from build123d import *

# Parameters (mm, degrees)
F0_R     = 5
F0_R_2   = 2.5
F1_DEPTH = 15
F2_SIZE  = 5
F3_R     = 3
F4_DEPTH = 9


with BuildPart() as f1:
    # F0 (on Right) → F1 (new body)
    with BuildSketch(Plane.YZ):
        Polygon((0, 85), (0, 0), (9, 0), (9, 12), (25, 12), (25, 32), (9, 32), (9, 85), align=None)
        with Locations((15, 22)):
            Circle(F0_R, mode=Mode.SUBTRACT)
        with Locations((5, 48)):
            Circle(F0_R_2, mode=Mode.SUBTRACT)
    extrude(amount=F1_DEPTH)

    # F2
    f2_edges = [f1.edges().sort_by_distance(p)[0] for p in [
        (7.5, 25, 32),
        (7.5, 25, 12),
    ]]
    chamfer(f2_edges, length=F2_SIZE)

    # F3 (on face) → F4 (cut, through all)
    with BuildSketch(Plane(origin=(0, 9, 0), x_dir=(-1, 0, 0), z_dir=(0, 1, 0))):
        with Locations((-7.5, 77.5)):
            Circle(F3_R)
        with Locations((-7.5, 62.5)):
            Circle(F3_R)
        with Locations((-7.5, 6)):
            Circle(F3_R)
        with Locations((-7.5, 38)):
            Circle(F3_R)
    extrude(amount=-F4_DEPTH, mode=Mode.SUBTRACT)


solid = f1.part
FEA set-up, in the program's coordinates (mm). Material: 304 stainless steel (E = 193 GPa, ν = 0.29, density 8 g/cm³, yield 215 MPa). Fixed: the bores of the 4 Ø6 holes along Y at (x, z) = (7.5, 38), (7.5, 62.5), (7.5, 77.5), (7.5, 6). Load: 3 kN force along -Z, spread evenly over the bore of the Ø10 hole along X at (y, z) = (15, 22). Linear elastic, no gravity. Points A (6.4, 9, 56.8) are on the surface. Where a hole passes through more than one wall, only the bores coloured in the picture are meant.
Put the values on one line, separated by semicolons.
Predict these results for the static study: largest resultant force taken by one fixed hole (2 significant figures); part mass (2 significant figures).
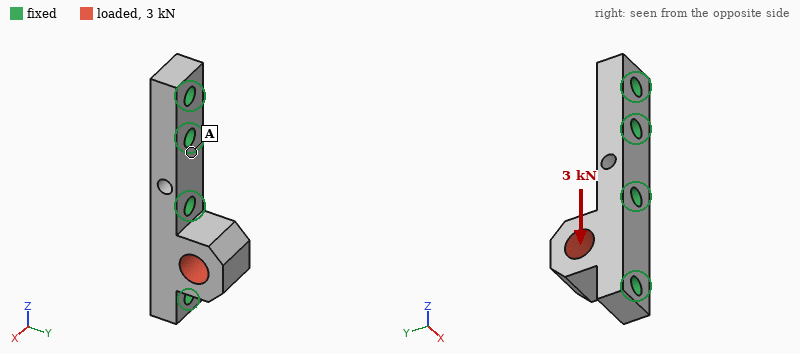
1.9 kN; 110 g
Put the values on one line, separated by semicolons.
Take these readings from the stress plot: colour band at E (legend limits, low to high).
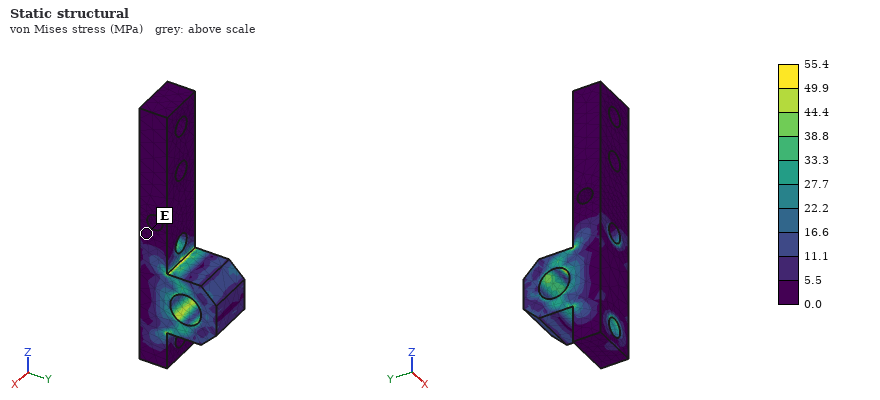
0.0 to 5.5 MPa
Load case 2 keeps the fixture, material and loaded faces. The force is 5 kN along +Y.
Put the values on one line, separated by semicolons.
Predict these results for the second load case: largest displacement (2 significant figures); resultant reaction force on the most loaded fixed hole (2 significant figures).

4.4 µm; 2.6 kN
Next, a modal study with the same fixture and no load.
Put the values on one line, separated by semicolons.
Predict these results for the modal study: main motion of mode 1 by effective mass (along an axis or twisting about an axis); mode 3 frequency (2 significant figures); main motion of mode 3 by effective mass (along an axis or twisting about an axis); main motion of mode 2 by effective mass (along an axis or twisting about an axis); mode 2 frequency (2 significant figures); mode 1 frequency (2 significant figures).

along X; 28 kHz; along Y; along Z; 21 kHz; 13 kHz
